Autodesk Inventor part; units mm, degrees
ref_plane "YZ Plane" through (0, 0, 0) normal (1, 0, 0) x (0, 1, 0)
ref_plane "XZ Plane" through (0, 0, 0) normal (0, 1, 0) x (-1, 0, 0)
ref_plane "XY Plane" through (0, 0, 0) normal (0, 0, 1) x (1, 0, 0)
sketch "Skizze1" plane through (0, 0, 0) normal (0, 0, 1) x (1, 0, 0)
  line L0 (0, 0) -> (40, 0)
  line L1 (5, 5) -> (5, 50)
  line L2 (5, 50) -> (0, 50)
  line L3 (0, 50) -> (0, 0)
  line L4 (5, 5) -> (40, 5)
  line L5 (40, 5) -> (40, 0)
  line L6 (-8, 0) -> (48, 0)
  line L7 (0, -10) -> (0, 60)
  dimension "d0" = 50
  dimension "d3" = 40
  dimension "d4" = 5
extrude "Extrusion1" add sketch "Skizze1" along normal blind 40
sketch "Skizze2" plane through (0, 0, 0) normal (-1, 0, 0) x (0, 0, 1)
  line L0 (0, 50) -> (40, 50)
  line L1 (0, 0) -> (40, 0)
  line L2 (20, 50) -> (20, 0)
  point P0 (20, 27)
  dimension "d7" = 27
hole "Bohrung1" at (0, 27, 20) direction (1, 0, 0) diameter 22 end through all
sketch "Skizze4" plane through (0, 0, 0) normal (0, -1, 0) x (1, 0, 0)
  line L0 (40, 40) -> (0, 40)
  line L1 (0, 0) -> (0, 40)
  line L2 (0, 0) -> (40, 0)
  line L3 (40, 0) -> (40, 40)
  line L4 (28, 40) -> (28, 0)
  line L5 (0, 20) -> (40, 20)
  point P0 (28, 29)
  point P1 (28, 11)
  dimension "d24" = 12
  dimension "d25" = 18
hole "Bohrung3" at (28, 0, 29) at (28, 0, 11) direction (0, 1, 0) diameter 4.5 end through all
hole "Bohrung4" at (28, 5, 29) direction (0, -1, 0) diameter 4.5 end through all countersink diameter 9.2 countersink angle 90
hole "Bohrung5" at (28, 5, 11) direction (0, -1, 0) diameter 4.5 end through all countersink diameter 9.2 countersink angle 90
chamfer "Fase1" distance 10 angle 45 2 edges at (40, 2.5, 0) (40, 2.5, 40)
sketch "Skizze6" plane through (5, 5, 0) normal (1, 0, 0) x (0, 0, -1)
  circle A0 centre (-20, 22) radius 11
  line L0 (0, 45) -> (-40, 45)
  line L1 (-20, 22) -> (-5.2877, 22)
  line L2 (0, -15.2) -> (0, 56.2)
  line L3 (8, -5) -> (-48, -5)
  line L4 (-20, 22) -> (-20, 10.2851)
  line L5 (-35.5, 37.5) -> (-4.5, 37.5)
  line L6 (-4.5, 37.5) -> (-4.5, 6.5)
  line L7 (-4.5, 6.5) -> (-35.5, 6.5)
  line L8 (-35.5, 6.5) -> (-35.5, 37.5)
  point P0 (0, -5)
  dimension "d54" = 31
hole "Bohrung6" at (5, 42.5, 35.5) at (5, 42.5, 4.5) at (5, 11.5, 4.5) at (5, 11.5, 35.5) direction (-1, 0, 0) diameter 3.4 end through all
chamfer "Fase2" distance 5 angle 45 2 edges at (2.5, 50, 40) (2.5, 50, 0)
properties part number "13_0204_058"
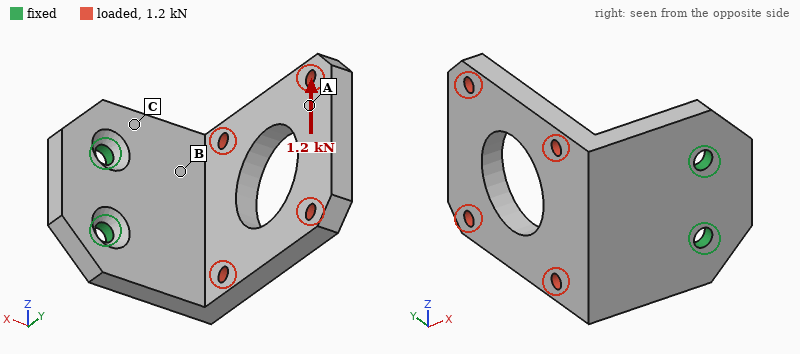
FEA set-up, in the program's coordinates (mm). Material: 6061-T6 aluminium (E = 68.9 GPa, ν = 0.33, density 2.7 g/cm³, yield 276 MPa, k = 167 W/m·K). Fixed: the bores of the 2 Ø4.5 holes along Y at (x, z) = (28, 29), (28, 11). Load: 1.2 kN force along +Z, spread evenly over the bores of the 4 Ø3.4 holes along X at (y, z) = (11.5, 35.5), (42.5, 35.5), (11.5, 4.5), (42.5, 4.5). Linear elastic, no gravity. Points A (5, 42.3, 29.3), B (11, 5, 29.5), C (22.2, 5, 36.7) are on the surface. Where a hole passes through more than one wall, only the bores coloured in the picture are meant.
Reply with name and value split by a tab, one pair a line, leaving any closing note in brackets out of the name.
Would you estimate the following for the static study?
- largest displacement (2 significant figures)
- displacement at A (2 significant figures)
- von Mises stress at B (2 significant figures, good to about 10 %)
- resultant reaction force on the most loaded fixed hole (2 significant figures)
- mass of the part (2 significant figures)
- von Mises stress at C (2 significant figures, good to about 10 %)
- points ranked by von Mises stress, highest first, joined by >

largest displacement	0.64 mm
displacement at A	0.53 mm
von Mises stress at B	120 MPa
resultant reaction force on the most loaded fixed hole	2.2 kN
mass of the part	38 g
von Mises stress at C	73 MPa
points ranked by von Mises stress, highest first, joined by >	B > C > A
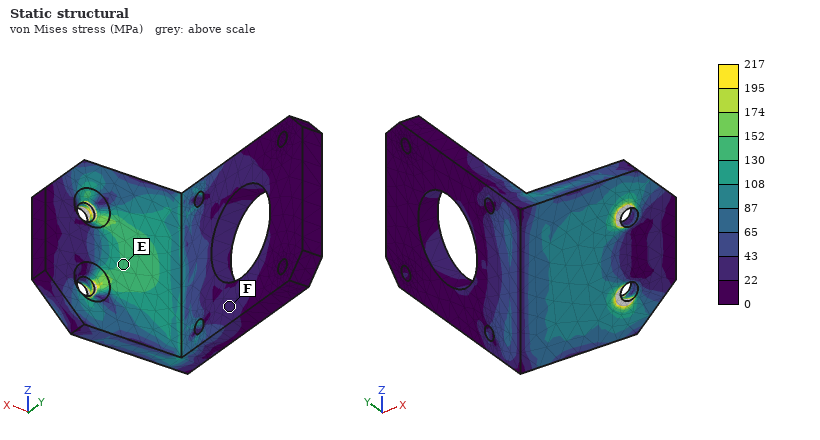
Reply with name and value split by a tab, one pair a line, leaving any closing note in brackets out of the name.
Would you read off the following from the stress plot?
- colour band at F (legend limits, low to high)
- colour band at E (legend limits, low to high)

colour band at F	22 to 43 MPa
colour band at E	130 to 152 MPa
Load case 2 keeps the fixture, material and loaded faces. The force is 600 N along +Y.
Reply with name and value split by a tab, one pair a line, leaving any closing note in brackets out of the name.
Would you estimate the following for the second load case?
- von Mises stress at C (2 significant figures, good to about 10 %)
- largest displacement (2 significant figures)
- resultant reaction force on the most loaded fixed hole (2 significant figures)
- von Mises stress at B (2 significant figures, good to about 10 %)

von Mises stress at C	67 MPa
largest displacement	0.48 mm
resultant reaction force on the most loaded fixed hole	310 N
von Mises stress at B	26 MPa
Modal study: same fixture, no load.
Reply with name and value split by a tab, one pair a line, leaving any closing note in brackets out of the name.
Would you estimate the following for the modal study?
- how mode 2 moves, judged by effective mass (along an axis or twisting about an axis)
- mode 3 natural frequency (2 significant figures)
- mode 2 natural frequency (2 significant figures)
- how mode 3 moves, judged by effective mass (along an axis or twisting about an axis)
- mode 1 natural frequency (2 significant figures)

how mode 2 moves, judged by effective mass	along Z
mode 3 natural frequency	2800 Hz
mode 2 natural frequency	1800 Hz
how mode 3 moves, judged by effective mass	along Y
mode 1 natural frequency	970 Hz
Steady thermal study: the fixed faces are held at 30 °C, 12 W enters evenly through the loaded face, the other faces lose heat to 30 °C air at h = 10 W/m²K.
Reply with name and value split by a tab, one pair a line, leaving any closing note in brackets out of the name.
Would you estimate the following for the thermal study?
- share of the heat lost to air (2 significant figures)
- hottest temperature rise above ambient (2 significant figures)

share of the heat lost to air	6.4 %
hottest temperature rise above ambient	23 K
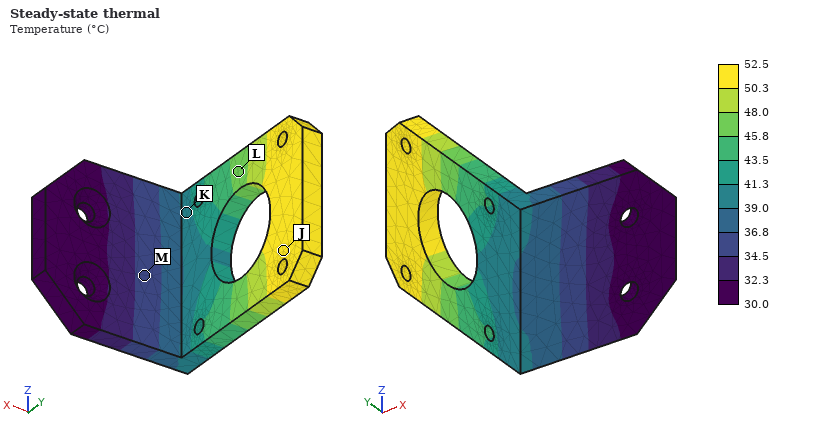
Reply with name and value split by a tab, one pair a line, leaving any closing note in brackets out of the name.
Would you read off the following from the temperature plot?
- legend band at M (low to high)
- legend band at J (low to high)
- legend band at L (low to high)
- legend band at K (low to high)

legend band at M	34.5 to 36.8 °C
legend band at J	50.3 to 52.5 °C
legend band at L	45.8 to 48.0 °C
legend band at K	39.0 to 41.3 °C
